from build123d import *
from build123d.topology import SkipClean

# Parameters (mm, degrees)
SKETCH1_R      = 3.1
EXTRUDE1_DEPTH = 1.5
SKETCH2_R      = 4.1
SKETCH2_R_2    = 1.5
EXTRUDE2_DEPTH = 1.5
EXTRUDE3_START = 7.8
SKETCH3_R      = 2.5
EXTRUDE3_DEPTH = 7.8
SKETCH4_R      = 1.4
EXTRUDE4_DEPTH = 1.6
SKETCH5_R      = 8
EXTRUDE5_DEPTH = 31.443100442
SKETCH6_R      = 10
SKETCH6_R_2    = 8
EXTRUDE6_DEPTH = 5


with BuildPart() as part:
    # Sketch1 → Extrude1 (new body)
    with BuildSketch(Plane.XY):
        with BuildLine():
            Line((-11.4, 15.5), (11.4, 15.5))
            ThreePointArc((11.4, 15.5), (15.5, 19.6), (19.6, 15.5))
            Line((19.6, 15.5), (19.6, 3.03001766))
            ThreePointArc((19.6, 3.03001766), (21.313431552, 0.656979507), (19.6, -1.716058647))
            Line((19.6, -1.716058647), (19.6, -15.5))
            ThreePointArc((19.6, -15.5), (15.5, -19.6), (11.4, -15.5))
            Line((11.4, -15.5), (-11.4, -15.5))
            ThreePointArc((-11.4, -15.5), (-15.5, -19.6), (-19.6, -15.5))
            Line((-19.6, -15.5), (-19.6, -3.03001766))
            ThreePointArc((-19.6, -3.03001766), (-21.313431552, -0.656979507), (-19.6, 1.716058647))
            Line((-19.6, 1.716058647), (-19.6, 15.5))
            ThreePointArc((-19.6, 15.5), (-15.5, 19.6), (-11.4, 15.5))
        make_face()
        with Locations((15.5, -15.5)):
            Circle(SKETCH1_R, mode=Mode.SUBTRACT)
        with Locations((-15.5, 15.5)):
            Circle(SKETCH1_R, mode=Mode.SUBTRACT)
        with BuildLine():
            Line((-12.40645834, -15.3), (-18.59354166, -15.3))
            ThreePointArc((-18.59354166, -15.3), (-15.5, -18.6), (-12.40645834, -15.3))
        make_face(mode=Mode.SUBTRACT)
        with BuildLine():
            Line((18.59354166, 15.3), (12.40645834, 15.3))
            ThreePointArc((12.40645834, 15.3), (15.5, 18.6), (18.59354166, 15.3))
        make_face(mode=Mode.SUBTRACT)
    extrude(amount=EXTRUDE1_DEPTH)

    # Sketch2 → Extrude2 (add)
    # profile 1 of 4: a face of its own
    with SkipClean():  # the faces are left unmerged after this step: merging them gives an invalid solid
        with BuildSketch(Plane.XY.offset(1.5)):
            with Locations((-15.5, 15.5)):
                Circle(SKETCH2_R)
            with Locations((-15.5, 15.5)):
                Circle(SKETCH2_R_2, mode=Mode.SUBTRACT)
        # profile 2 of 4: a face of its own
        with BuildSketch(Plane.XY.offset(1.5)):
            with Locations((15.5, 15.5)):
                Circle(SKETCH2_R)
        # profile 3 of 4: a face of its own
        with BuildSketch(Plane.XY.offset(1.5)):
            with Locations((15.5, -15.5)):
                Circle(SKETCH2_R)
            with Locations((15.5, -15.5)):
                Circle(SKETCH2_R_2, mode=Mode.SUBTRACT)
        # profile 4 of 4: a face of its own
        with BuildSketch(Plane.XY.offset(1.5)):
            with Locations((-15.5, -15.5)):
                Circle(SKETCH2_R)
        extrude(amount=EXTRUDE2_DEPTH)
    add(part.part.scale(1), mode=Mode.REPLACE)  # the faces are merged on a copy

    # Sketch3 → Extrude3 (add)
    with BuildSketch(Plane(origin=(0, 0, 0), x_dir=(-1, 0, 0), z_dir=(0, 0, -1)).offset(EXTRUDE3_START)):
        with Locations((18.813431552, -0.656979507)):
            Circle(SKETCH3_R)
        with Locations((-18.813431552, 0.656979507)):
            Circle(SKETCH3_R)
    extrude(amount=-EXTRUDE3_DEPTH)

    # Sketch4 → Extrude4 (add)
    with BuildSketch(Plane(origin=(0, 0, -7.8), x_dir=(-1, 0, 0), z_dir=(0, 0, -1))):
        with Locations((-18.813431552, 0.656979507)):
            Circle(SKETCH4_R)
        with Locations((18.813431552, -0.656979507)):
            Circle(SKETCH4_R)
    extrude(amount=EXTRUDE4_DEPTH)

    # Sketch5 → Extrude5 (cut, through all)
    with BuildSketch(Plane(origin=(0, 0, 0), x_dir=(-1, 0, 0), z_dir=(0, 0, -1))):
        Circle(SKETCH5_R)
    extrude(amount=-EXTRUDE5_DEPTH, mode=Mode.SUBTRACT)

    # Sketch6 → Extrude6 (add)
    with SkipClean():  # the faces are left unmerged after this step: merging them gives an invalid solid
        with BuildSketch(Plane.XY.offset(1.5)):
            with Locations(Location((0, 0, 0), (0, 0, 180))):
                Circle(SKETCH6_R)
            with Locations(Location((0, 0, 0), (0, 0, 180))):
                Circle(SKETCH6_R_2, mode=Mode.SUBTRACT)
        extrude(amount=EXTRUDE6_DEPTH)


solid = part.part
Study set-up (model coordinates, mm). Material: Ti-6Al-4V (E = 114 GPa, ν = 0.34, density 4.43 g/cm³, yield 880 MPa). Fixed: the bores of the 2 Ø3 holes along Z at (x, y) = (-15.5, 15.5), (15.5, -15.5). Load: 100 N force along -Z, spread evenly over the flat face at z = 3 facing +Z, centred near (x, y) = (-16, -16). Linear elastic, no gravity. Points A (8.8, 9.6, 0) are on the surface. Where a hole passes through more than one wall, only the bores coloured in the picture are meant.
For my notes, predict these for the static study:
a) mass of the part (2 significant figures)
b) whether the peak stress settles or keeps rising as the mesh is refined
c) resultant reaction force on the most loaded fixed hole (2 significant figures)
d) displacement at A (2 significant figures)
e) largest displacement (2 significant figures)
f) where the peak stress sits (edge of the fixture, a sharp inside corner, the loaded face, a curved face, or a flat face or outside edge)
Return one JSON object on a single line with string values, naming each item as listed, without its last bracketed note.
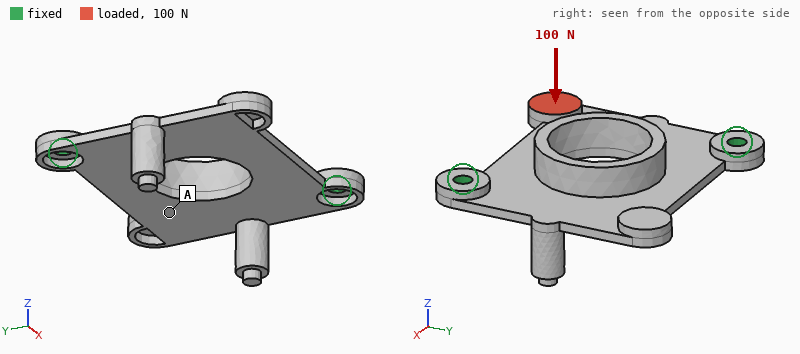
{"mass of the part": "12 g", "whether the peak stress settles or keeps rising as the mesh is refined": "keeps rising", "resultant reaction force on the most loaded fixed hole": "60 N", "displacement at A": "0.14 mm", "largest displacement": "0.64 mm", "where the peak stress sits": "edge of the fixture"}
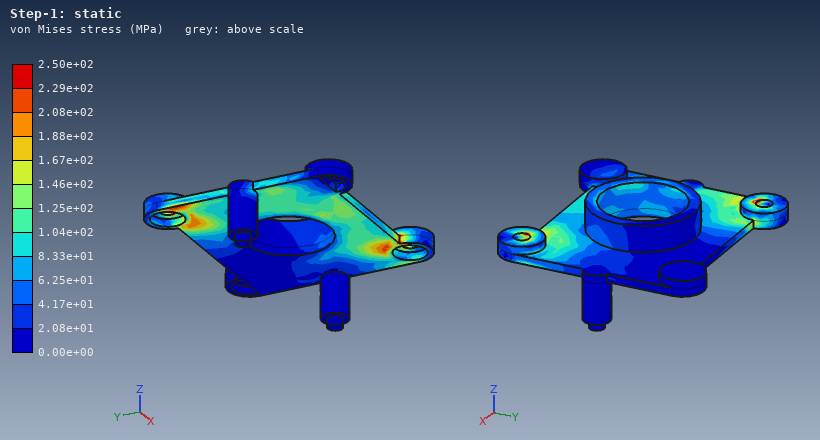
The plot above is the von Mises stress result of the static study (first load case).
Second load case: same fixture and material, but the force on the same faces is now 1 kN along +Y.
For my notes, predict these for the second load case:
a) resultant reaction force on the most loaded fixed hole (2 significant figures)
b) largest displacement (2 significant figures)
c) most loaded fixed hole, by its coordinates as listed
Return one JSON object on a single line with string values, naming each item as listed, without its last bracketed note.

{"resultant reaction force on the most loaded fixed hole": "900 N", "largest displacement": "0.70 mm", "most loaded fixed hole, by its coordinates as listed": "(-15.5, 15.5)"}
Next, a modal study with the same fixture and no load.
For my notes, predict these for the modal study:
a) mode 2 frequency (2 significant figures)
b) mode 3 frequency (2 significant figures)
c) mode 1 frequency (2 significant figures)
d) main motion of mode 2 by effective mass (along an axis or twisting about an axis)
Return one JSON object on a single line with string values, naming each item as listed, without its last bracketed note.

{"mode 2 frequency": "2700 Hz", "mode 3 frequency": "5900 Hz", "mode 1 frequency": "1500 Hz", "main motion of mode 2 by effective mass": "along Z"}
